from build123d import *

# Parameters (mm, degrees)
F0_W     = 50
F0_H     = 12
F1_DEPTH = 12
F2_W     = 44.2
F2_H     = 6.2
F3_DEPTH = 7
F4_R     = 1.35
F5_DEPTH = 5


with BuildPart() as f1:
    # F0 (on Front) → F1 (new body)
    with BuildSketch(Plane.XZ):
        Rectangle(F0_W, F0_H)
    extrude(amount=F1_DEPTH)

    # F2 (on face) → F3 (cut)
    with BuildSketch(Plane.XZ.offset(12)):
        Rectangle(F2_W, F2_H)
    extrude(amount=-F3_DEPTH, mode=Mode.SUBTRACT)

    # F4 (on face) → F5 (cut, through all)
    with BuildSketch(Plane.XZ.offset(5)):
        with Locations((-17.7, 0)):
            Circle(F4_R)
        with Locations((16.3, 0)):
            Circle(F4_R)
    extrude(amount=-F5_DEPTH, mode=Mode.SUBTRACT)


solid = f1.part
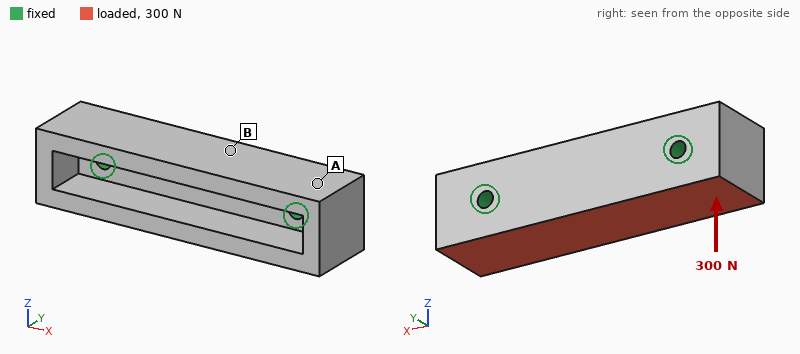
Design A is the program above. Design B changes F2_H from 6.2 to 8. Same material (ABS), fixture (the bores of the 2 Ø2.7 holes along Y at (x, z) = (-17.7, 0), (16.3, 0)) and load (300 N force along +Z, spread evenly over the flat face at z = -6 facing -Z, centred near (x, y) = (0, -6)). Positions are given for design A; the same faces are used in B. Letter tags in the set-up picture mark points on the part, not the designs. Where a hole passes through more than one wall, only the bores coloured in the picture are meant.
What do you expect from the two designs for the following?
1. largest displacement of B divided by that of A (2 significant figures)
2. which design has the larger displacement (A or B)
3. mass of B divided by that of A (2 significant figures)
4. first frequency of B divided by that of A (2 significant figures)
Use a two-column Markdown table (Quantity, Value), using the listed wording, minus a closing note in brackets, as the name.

| Quantity | Value |
|---|---|
| largest displacement of B divided by that of A | 1.6 |
| which design has the larger displacement | B |
| mass of B divided by that of A | 0.89 |
| first frequency of B divided by that of A | 1.0 |
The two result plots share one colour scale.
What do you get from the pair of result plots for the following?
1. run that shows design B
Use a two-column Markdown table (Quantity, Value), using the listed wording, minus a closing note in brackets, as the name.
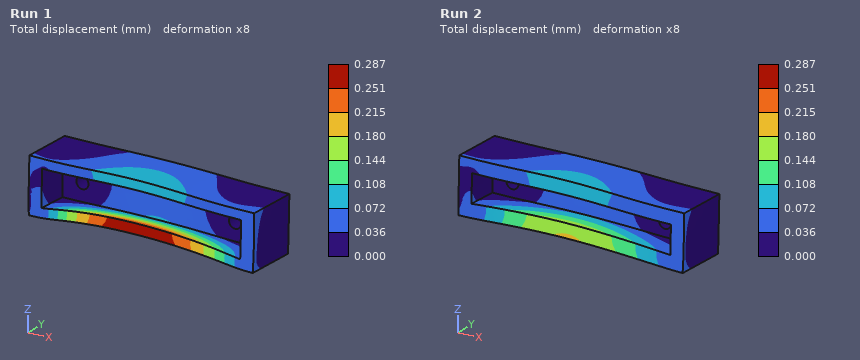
| Quantity | Value |
|---|---|
| run that shows design B | Run 1 |
